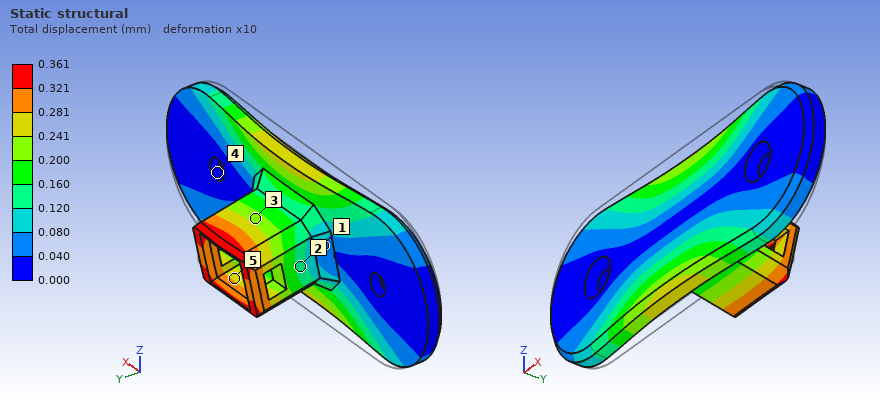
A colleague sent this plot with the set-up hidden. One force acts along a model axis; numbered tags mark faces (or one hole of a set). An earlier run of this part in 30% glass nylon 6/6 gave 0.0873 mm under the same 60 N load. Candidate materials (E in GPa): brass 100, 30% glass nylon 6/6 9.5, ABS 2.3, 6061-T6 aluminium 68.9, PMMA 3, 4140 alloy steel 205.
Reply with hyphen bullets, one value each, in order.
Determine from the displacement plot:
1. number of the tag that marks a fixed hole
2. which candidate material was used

- 4
- ABS
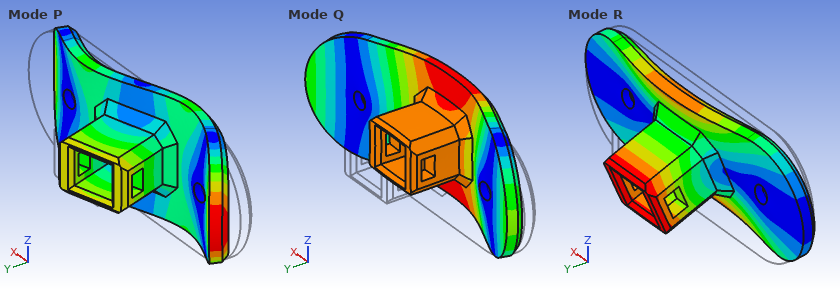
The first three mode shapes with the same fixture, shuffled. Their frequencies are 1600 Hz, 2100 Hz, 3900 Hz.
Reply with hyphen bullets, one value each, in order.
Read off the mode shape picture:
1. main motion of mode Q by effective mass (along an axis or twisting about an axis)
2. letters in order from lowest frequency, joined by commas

- along Y
- R, Q, P
